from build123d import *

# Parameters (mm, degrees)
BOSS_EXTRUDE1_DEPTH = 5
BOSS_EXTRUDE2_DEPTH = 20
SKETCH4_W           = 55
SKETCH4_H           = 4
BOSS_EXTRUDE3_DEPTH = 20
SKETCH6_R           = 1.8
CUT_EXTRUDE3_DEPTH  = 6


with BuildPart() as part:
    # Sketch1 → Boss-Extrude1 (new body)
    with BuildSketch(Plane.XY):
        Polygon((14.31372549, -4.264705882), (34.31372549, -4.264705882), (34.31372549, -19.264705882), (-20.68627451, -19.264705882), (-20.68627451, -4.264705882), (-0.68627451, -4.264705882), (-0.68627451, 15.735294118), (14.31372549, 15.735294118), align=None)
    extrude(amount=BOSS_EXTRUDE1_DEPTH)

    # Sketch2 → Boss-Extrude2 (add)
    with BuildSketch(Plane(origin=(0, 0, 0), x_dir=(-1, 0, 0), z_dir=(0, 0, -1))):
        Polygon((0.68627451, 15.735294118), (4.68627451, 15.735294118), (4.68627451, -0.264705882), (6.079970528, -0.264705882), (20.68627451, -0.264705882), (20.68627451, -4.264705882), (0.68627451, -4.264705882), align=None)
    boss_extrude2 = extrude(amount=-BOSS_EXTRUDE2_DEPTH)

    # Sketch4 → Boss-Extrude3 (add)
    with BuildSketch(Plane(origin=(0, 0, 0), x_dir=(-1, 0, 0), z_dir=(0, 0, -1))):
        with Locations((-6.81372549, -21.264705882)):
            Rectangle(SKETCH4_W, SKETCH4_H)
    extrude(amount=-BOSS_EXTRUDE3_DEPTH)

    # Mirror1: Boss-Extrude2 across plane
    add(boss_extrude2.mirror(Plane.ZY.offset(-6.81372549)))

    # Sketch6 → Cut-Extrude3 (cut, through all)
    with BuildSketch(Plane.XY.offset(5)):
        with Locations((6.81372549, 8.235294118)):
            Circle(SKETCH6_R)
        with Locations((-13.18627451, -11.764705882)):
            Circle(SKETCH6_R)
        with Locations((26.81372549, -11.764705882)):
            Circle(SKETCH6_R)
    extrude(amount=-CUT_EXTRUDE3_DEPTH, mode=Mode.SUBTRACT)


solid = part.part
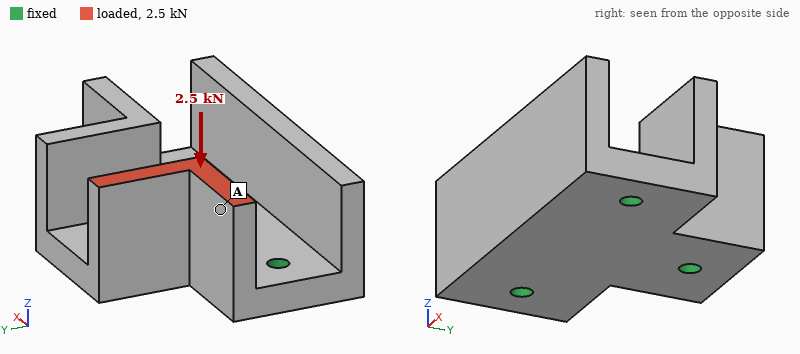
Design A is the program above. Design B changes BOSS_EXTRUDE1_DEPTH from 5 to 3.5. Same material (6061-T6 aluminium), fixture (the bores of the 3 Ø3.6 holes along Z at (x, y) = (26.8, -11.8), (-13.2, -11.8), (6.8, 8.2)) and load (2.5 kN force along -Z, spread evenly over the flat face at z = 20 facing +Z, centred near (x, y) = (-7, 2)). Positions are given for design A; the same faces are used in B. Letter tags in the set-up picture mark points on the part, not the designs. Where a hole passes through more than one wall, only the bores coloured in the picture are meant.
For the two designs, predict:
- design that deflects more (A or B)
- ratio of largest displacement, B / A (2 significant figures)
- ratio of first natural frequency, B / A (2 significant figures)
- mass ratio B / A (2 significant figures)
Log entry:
B
2.1
0.64
0.89
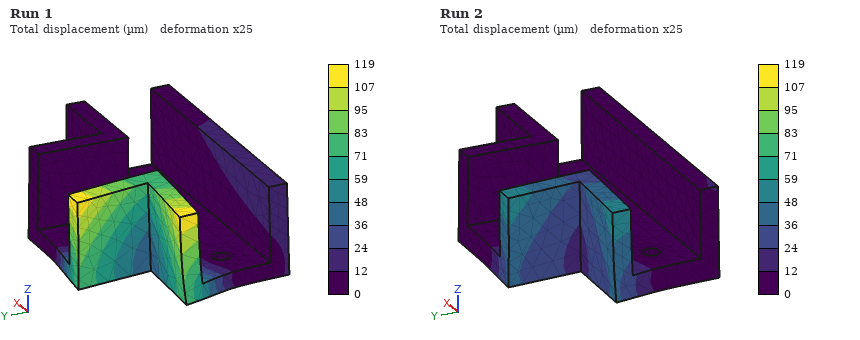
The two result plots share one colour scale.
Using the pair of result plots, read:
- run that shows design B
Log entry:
Run 1
